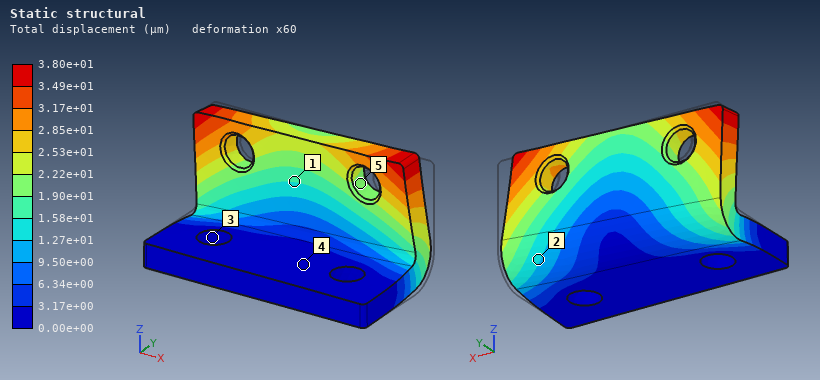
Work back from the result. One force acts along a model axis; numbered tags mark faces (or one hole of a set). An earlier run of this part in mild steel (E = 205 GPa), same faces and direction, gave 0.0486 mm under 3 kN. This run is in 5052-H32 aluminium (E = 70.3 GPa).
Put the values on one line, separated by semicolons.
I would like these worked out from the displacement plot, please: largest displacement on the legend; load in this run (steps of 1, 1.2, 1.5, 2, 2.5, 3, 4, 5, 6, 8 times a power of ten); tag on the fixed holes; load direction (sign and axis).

3.80e+01 µm; 800 N; 3; -X
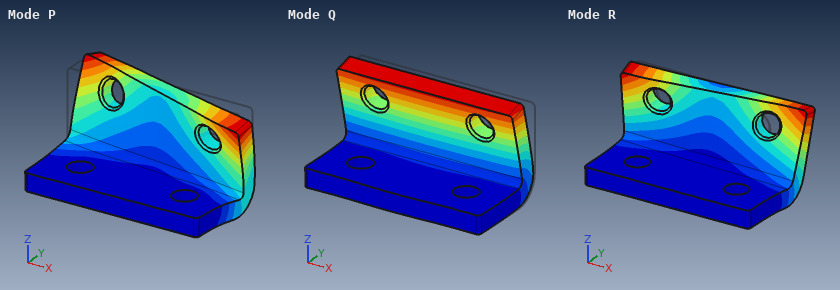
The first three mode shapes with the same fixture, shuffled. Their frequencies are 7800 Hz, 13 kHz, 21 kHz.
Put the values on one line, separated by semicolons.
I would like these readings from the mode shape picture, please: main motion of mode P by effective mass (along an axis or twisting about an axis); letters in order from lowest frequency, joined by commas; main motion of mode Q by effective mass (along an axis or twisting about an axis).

along X; Q, R, P; along Y
